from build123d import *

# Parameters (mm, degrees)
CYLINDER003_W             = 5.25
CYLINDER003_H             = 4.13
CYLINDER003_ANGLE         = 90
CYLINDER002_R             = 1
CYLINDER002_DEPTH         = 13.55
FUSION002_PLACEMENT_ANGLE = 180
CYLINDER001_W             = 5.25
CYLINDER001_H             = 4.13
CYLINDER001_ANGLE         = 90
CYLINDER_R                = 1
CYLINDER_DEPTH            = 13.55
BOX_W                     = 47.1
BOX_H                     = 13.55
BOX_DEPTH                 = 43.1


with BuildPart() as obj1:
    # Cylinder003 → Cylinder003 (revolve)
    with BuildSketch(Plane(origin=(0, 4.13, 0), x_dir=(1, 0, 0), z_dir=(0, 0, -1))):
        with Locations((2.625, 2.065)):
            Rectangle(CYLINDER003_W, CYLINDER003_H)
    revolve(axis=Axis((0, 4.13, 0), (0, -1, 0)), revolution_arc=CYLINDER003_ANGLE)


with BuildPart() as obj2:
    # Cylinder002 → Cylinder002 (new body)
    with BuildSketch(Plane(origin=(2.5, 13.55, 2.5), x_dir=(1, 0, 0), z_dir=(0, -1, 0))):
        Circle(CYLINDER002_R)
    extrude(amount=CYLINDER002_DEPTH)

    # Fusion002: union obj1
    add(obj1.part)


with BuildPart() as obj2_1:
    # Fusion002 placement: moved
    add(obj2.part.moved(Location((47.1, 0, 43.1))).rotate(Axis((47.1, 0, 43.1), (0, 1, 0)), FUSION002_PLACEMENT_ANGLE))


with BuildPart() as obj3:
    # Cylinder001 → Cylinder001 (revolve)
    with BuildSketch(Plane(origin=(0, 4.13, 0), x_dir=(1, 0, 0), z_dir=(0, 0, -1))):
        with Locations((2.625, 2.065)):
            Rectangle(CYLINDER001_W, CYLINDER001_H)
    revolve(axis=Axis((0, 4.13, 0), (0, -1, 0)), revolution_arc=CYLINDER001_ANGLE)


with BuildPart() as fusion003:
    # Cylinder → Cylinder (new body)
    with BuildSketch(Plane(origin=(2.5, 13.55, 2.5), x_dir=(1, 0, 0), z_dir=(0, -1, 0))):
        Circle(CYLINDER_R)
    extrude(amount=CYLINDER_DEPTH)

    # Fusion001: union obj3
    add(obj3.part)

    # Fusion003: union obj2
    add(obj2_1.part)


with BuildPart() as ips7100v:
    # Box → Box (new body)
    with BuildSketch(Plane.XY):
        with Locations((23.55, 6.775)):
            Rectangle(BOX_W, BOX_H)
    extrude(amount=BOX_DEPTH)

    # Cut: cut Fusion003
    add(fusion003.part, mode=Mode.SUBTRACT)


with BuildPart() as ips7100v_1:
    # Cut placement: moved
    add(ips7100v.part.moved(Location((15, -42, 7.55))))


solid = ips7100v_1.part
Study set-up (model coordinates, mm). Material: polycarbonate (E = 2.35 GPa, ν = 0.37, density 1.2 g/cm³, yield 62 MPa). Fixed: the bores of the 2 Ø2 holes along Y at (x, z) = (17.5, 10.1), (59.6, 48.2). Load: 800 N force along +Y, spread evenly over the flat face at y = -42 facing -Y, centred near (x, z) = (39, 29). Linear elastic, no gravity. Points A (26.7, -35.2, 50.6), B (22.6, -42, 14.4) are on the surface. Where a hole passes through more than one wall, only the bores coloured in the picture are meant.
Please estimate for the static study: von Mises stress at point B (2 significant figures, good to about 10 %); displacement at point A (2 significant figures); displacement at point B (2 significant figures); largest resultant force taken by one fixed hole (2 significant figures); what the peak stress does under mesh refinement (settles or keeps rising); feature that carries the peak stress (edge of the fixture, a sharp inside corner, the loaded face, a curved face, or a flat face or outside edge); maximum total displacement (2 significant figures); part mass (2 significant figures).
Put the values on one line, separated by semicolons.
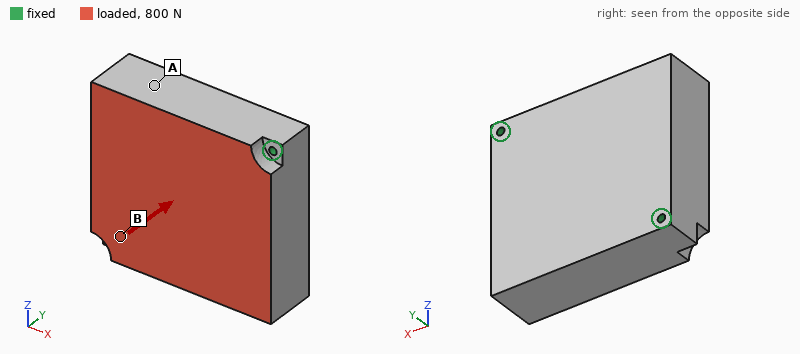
3.9 MPa; 0.18 mm; 0.072 mm; 440 N; keeps rising; edge of the fixture; 0.21 mm; 33 g
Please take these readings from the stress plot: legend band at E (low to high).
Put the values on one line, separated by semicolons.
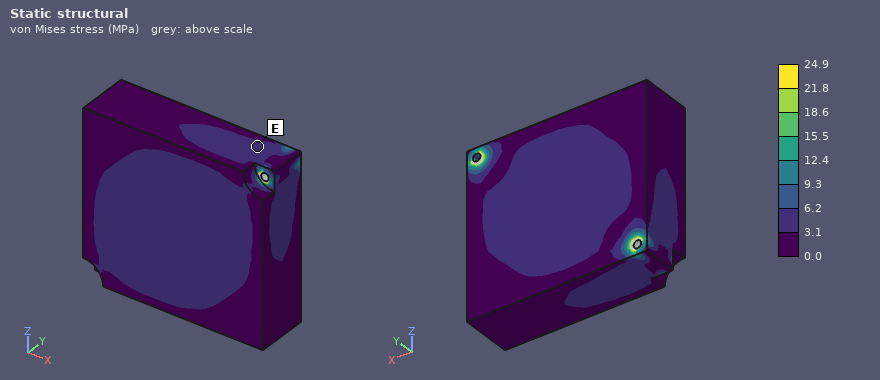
3.1 to 6.2 MPa
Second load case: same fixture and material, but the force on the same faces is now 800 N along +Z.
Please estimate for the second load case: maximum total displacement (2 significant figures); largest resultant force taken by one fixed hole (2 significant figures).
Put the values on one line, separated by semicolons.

0.47 mm; 410 N
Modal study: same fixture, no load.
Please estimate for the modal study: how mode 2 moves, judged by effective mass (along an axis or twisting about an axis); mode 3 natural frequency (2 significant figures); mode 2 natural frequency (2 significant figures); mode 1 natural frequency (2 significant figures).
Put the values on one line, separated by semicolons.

along Y; 3600 Hz; 2100 Hz; 1200 Hz
